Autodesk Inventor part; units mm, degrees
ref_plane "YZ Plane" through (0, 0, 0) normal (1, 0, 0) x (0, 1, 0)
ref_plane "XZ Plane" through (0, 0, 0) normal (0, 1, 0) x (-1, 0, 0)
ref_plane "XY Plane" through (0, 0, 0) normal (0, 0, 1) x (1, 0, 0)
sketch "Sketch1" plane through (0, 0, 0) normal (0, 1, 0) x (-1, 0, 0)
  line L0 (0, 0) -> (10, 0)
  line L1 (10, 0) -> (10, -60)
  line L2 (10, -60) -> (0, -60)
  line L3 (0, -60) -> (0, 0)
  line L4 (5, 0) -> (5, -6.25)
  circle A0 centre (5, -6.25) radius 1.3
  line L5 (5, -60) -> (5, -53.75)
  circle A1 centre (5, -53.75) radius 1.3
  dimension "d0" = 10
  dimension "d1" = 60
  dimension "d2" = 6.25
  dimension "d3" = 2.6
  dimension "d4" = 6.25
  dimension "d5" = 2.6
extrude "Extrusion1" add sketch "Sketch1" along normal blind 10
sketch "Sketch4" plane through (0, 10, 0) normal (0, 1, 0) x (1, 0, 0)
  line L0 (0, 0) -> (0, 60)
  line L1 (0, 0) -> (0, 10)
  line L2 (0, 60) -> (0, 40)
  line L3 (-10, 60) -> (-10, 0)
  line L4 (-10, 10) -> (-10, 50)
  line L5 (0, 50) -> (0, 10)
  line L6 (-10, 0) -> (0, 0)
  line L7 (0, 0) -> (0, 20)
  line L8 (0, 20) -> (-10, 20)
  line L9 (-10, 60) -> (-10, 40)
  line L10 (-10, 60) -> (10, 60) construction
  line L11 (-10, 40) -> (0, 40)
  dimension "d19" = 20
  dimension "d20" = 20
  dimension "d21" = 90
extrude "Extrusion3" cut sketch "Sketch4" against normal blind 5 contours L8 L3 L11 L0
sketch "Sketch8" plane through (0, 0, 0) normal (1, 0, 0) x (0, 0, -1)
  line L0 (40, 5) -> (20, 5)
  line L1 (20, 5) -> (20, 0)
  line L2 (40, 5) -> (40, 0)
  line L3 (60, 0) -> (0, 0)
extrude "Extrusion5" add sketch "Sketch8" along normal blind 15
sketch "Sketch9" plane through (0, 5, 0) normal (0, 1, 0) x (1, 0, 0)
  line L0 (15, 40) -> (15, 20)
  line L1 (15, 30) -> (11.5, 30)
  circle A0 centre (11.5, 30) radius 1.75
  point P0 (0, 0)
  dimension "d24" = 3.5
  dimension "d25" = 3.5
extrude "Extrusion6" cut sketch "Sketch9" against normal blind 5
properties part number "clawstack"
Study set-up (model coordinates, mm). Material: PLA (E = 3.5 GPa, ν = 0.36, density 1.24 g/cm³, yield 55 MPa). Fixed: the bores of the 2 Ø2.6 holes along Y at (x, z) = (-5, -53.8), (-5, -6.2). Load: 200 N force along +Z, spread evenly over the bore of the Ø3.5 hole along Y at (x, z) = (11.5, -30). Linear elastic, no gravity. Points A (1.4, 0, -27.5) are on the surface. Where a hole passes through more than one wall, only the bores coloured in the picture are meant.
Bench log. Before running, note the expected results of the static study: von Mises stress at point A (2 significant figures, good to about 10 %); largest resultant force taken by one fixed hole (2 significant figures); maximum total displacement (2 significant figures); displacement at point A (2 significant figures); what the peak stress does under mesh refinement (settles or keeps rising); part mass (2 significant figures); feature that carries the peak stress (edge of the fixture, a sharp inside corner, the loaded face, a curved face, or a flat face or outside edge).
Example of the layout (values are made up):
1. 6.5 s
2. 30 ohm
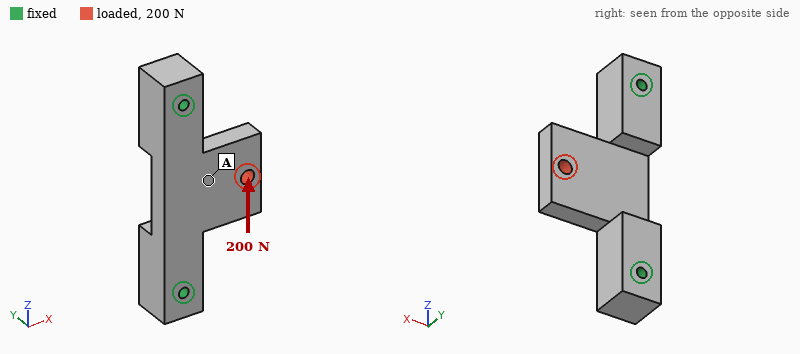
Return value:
1. 2.0 MPa
2. 130 N
3. 0.11 mm
4. 0.024 mm
5. keeps rising
6. 7.9 g
7. a sharp inside corner
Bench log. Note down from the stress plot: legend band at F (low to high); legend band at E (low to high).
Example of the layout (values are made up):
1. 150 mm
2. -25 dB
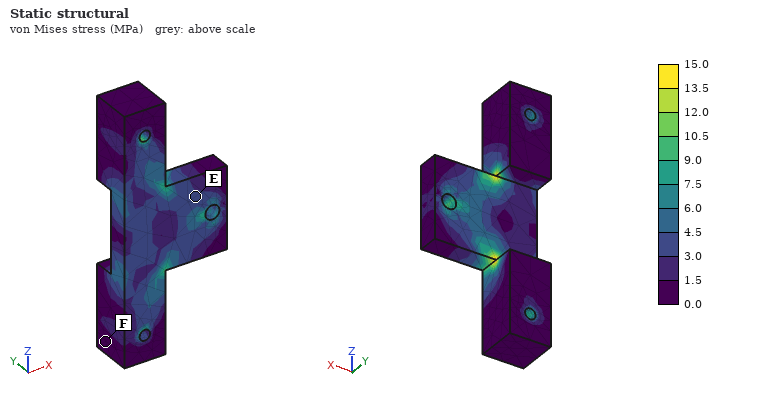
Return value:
1. 0.0 to 1.5 MPa
2. 3.0 to 4.5 MPa
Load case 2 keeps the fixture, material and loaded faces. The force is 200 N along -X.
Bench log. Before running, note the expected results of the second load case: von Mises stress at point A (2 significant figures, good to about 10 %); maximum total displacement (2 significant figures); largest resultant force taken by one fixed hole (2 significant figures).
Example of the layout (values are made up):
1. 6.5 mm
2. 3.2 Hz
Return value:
1. 2.2 MPa
2. 0.10 mm
3. 110 N
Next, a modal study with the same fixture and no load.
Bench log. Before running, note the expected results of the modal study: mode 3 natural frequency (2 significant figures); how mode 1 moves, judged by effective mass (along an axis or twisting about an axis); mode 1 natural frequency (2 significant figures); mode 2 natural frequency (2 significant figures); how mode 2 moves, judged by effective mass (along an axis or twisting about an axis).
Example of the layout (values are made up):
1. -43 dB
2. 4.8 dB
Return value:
1. 6100 Hz
2. along Y
3. 2400 Hz
4. 4400 Hz
5. along X
